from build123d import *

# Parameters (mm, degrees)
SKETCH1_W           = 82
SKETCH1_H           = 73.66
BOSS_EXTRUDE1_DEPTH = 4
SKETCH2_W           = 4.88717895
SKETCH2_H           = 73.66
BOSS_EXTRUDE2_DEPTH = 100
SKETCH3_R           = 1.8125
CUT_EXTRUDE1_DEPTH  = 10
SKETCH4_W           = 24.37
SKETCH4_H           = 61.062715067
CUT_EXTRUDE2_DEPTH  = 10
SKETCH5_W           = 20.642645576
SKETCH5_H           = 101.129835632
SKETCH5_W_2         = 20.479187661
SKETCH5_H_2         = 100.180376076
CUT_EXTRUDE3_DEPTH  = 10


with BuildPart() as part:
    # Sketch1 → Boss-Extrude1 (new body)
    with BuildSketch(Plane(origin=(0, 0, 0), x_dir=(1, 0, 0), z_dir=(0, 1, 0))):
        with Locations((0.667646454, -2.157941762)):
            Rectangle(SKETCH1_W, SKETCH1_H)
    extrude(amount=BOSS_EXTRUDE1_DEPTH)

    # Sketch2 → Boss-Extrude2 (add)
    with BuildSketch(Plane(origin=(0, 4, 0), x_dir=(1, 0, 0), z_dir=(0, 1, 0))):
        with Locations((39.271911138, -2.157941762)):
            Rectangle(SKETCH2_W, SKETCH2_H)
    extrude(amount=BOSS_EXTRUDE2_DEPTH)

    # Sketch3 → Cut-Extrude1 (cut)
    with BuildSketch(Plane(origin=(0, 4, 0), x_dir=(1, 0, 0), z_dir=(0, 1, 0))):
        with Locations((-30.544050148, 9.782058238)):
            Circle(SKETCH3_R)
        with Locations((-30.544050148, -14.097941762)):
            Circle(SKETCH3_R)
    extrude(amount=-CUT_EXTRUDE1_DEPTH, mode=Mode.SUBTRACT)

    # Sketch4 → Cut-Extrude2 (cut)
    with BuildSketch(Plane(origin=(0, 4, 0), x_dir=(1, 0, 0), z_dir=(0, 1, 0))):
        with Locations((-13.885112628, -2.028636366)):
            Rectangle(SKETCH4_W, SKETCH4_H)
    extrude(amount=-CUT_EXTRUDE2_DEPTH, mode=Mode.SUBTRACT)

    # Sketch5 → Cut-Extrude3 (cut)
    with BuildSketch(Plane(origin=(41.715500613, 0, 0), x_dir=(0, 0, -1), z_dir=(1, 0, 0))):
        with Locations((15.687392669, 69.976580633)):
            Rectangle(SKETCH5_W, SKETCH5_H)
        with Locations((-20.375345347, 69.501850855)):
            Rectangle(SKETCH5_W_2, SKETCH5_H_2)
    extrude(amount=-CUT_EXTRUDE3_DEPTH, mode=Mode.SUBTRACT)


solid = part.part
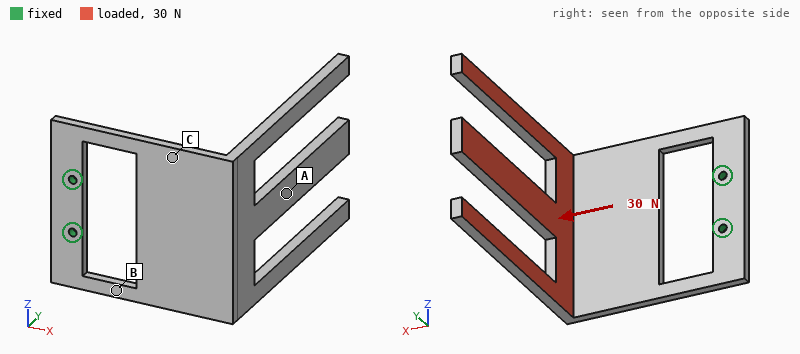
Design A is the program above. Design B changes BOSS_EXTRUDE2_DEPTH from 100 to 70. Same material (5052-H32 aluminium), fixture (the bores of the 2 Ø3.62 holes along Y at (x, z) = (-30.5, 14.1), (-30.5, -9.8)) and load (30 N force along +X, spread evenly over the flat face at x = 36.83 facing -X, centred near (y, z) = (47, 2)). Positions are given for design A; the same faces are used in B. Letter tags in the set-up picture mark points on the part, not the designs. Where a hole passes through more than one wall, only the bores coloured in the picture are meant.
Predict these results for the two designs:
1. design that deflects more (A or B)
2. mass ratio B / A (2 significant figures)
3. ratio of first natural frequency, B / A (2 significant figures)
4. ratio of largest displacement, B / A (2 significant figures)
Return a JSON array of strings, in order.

["A", "0.87", "1.3", "0.52"]
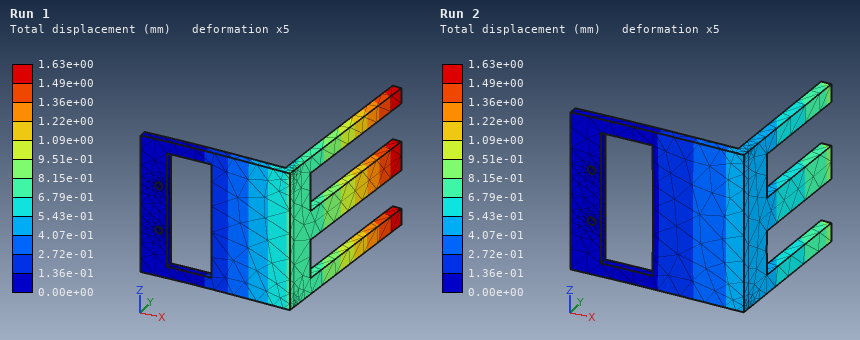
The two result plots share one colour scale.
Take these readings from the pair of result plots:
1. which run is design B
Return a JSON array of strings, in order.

["Run 2"]
